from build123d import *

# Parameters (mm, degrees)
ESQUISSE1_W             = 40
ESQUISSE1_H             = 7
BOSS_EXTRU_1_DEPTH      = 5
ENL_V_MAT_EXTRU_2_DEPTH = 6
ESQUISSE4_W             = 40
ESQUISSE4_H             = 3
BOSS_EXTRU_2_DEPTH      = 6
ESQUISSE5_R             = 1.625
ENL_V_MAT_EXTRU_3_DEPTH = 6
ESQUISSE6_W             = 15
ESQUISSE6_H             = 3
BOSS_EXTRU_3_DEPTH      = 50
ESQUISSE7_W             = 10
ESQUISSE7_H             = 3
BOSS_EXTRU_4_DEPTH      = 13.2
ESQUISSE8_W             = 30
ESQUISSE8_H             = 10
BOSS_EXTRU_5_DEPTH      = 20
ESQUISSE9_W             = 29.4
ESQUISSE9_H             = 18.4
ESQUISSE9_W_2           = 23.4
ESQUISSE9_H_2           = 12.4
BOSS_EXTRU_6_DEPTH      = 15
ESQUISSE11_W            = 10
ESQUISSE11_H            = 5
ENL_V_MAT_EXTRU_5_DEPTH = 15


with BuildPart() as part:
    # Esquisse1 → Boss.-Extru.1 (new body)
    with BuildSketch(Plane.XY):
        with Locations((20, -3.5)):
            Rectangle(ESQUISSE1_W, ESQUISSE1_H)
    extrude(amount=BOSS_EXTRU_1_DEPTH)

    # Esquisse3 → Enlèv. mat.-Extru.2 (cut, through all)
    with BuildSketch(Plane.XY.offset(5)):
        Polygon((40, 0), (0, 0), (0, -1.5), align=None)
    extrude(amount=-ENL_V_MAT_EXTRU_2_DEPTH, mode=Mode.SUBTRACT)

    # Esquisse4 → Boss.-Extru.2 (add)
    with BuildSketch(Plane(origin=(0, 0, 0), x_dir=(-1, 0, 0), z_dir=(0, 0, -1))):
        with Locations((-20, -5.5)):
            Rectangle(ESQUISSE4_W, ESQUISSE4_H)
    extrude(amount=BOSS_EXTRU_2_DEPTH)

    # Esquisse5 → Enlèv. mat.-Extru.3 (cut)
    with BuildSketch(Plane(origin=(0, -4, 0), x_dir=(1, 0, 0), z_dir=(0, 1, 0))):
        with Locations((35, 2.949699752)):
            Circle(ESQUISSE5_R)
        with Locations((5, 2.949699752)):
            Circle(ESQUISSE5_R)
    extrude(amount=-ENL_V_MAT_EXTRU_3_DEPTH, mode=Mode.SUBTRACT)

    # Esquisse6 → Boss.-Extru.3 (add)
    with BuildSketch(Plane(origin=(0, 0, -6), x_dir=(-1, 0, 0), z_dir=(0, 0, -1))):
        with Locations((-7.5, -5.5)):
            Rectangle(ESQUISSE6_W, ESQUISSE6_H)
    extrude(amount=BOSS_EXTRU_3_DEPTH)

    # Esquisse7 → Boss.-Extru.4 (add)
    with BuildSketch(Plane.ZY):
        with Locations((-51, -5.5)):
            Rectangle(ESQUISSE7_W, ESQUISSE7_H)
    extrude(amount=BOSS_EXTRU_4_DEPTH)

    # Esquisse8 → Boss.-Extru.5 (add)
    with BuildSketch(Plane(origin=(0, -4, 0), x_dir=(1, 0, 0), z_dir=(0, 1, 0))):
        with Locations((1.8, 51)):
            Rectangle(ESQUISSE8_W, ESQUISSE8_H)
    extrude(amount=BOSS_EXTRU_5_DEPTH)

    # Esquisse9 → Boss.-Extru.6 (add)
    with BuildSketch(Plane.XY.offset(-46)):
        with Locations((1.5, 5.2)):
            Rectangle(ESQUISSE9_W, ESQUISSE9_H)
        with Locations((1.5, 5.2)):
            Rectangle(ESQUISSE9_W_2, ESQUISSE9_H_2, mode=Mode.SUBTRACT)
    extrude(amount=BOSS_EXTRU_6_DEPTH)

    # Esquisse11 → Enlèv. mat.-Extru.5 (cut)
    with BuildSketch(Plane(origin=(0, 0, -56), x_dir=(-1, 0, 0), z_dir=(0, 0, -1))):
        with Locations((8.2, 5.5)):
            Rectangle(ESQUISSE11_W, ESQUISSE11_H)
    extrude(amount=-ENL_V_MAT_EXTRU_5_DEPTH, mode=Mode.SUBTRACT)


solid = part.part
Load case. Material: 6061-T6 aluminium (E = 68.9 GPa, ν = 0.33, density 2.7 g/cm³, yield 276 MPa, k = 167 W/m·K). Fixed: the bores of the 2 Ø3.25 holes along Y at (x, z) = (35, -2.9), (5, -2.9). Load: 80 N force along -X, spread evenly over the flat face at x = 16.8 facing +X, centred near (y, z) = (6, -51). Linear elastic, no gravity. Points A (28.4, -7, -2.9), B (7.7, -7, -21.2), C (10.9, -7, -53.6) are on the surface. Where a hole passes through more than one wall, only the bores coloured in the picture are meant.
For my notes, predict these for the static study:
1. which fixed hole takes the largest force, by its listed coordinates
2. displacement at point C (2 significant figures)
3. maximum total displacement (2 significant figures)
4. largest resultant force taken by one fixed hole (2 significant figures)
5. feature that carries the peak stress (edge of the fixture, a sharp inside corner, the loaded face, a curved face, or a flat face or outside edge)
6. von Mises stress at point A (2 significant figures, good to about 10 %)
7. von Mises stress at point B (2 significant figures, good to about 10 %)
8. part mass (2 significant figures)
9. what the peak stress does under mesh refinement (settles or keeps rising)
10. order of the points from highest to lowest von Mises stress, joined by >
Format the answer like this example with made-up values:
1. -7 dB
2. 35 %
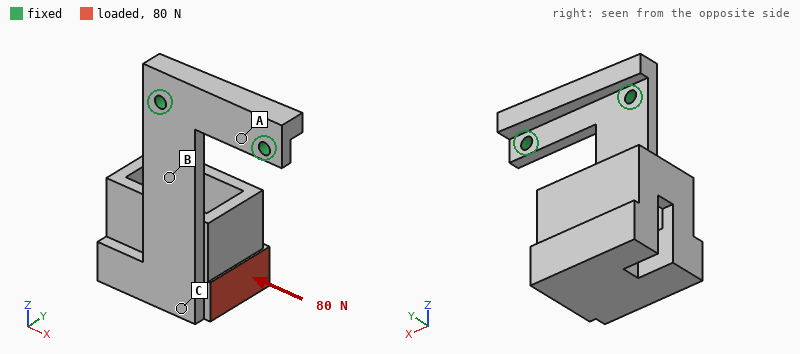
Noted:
1. (5, -2.9)
2. 0.074 mm
3. 0.28 mm
4. 180 N
5. edge of the fixture
6. 11 MPa
7. 31 MPa
8. 37 g
9. keeps rising
10. B > A > C
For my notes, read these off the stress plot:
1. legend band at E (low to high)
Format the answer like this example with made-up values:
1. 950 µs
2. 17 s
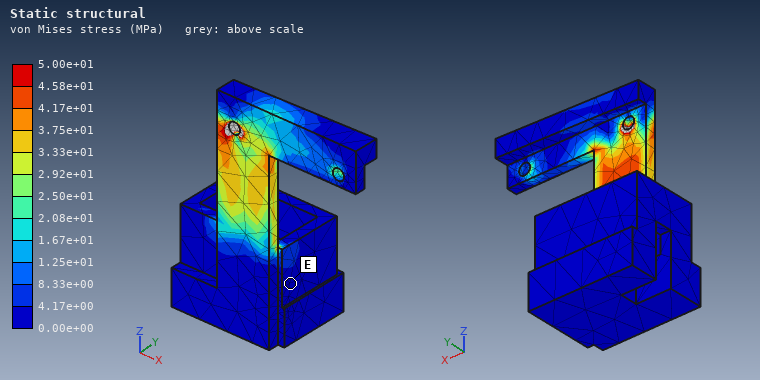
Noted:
1. 0.00e+00 to 4.17e+00 MPa
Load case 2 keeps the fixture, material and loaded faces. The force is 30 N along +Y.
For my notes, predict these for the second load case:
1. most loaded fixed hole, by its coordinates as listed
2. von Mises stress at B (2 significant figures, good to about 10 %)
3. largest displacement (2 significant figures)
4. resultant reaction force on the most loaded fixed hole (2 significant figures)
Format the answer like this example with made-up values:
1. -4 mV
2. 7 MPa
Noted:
1. (5, -2.9)
2. 40 MPa
3. 0.59 mm
4. 35 N
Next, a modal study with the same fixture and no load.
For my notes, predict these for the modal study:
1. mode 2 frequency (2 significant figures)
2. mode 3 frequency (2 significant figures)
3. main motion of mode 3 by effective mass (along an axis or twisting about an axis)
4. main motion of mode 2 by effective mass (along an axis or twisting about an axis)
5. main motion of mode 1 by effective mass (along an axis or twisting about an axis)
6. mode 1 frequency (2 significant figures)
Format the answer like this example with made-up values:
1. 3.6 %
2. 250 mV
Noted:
1. 630 Hz
2. 1500 Hz
3. along X
4. along X
5. along Y
6. 260 Hz
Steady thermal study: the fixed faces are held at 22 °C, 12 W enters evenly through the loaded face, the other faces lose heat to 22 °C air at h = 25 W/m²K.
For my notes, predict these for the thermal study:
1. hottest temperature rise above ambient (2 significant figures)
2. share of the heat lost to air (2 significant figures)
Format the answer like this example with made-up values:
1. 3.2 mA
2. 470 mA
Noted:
1. 39 K
2. 39 %
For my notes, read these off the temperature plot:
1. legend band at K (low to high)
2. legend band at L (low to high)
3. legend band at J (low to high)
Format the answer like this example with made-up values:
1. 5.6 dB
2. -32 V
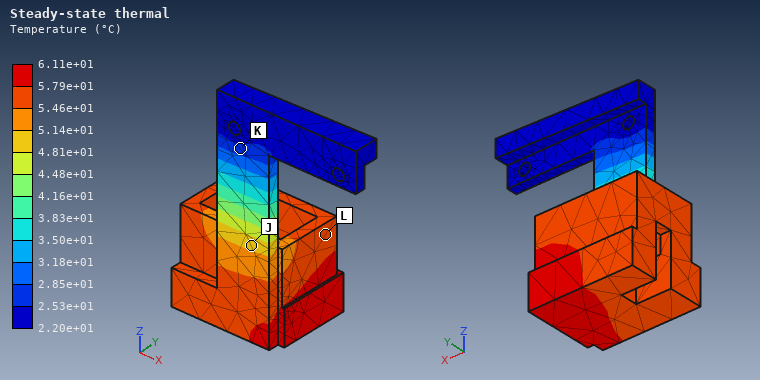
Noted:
1. 2.53e+01 to 2.85e+01 °C
2. 5.46e+01 to 5.79e+01 °C
3. 4.81e+01 to 5.14e+01 °C
